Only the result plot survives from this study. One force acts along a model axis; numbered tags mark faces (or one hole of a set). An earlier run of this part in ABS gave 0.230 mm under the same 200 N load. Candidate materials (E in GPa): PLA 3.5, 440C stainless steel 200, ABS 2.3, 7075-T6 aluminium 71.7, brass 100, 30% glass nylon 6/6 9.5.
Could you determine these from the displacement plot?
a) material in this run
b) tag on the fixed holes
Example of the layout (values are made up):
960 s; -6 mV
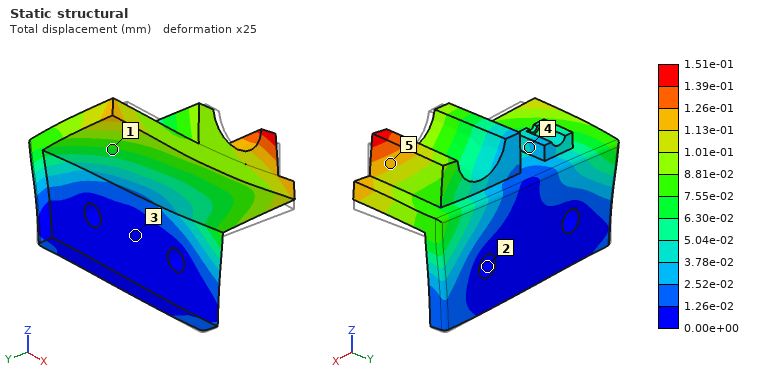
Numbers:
PLA; 2
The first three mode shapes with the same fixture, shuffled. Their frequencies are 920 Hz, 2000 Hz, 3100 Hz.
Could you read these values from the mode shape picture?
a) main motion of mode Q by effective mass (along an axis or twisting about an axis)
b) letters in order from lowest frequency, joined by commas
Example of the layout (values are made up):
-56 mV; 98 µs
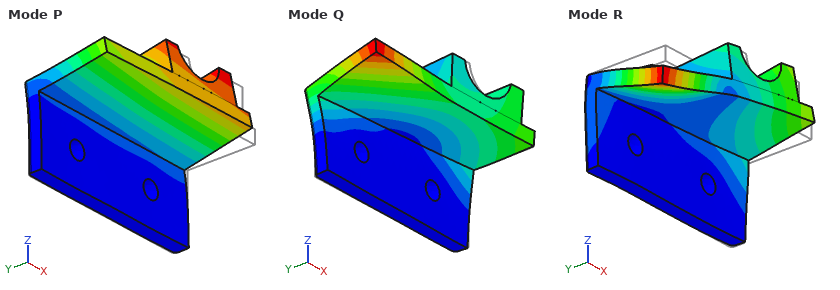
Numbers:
along X; P, Q, R
